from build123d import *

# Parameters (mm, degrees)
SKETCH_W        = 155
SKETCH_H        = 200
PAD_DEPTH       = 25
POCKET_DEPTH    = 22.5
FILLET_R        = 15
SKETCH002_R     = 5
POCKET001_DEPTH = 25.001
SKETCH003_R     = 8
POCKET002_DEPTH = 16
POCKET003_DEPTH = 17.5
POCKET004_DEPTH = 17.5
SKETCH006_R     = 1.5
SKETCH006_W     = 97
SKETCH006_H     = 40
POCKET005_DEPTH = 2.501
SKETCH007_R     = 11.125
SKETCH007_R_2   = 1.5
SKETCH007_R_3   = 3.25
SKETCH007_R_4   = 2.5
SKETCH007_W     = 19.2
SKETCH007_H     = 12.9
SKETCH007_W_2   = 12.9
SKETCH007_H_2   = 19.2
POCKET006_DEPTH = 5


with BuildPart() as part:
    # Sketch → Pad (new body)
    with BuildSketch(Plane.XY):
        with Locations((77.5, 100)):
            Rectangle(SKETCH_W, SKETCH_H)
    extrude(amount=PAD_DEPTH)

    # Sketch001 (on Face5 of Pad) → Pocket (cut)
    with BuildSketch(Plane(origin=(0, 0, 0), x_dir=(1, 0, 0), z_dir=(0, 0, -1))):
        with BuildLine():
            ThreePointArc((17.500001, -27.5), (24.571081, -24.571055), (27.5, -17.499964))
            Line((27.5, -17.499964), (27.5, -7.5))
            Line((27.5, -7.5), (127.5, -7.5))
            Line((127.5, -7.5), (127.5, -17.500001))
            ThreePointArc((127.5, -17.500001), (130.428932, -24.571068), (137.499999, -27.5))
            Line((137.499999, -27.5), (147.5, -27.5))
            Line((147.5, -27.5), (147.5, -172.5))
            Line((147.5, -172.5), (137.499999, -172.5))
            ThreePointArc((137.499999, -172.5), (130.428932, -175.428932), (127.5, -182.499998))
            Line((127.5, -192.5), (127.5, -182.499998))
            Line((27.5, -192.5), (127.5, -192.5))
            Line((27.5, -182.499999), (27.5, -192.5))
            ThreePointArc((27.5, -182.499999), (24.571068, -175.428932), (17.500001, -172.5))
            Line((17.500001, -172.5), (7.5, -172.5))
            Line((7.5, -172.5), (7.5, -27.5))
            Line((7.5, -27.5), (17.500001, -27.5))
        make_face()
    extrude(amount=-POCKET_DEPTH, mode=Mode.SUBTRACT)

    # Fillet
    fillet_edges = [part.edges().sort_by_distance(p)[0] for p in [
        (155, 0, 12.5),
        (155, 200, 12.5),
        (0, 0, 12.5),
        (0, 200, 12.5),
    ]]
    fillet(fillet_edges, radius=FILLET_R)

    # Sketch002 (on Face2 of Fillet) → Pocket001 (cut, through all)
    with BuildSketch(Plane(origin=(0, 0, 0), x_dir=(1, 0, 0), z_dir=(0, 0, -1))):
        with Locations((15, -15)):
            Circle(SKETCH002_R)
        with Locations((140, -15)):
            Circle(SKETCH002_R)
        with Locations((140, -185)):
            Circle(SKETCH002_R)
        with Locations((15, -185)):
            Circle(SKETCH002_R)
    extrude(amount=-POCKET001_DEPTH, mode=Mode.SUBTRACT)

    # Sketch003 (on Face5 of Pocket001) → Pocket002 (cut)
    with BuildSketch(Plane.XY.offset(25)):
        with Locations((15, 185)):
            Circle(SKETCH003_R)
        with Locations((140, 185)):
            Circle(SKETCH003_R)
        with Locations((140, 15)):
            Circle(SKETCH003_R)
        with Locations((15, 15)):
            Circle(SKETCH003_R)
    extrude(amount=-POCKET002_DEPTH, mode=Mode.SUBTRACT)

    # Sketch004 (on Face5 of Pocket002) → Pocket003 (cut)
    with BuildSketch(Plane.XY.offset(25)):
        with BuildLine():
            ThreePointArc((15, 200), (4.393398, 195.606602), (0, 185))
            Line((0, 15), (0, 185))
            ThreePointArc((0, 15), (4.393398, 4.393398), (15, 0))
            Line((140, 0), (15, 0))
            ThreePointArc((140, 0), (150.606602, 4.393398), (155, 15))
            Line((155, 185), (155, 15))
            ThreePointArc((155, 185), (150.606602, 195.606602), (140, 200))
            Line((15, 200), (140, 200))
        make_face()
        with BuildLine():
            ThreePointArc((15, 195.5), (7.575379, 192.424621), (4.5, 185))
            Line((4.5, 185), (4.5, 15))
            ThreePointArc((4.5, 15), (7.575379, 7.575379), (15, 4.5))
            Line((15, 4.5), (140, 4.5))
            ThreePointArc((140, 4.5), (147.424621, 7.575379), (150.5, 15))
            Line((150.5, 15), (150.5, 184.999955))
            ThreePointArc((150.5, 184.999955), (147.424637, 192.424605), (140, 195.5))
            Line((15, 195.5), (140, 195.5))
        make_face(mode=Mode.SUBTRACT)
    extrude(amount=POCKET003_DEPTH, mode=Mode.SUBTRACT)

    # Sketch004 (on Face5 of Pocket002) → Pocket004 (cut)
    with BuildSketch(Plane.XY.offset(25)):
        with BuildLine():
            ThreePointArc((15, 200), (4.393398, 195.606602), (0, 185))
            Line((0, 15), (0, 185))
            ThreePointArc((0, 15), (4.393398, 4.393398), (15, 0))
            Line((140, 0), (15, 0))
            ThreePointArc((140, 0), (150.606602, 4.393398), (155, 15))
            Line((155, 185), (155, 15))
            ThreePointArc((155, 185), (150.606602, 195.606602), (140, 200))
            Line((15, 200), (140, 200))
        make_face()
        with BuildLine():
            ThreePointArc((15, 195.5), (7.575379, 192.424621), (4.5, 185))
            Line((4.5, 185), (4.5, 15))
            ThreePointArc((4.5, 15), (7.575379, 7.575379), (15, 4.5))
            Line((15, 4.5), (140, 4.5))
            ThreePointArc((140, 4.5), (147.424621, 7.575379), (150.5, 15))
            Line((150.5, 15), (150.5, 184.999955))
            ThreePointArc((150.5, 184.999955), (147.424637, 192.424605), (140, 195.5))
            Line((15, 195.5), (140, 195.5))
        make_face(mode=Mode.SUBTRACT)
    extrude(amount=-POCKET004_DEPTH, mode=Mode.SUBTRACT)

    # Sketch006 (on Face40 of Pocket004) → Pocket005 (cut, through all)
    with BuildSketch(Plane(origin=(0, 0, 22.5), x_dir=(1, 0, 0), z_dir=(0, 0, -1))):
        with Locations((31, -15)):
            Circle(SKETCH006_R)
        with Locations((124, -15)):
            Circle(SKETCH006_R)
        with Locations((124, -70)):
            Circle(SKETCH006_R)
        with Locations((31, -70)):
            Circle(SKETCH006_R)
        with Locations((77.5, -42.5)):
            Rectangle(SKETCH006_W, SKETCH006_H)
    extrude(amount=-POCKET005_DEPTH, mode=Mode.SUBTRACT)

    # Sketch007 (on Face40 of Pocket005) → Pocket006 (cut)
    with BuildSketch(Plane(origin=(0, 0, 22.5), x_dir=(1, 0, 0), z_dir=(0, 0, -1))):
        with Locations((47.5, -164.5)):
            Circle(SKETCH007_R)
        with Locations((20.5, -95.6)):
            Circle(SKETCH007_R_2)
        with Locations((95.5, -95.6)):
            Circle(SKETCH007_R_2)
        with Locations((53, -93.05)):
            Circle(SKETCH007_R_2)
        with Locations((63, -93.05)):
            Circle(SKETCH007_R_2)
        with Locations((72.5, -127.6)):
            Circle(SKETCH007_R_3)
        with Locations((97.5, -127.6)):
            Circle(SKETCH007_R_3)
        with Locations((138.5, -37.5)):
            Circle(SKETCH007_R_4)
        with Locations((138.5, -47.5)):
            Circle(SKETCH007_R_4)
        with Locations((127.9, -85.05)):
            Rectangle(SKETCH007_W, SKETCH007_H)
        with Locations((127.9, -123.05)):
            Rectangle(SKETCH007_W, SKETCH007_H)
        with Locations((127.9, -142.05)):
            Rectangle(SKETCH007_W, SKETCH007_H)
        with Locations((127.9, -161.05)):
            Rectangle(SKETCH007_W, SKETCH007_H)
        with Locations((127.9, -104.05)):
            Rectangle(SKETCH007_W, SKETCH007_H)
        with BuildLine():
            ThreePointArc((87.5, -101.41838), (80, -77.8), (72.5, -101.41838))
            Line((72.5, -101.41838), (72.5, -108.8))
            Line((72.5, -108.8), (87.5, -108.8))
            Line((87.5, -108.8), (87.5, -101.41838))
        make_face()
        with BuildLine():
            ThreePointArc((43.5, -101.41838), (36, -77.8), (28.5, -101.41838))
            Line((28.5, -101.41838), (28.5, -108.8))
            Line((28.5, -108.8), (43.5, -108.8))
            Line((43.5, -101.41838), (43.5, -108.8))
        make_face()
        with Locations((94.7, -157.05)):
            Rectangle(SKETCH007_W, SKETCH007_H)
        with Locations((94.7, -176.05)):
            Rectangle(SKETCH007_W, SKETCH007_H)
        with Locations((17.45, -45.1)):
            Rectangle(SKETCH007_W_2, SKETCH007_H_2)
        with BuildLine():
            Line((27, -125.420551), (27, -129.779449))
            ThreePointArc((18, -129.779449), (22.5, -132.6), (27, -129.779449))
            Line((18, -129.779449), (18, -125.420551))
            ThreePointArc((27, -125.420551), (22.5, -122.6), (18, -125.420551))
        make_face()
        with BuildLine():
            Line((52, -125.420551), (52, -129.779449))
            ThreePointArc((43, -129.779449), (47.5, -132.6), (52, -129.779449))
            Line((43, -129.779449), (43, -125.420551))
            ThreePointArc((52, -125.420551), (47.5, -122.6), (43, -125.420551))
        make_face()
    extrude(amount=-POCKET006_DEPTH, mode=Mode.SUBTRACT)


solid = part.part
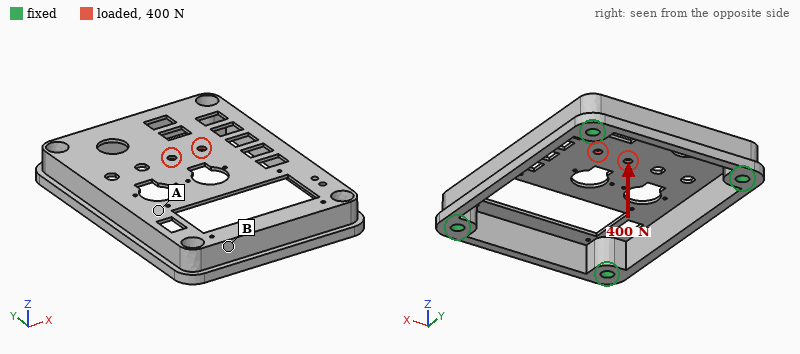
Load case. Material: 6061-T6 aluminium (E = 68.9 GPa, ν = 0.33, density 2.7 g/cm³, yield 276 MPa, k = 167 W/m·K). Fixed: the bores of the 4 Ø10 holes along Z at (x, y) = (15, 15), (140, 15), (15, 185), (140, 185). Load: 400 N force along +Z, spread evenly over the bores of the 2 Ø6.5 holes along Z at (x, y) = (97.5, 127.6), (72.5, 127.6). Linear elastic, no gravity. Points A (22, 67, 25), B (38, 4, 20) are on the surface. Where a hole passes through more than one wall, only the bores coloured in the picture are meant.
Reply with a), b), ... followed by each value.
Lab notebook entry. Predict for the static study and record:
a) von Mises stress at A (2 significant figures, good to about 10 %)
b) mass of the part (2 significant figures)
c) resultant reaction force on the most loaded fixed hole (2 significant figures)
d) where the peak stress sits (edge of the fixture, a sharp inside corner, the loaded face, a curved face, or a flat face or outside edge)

a) 22 MPa
b) 360 g
c) 210 N
d) the loaded face
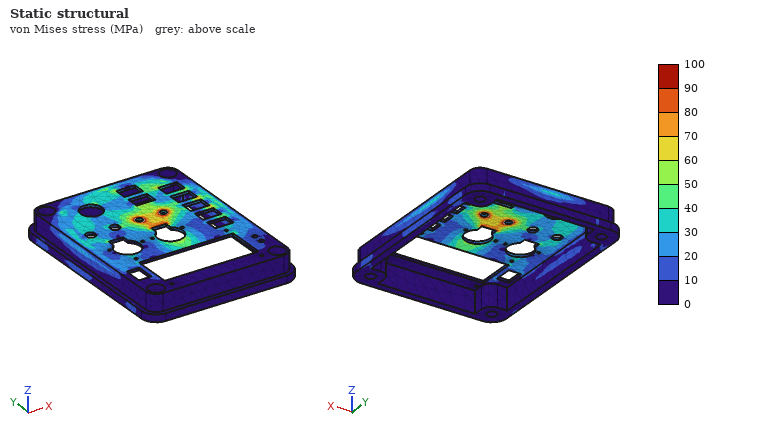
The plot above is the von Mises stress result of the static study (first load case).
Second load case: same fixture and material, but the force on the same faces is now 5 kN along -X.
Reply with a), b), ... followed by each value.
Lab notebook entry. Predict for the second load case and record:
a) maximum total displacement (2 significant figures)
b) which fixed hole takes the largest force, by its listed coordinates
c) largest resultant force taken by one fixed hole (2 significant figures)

a) 0.11 mm
b) (15, 185)
c) 2.5 kN
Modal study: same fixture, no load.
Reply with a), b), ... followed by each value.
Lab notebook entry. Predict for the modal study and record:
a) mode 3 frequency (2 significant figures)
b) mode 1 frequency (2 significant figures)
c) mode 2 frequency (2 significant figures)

a) 1600 Hz
b) 650 Hz
c) 1200 Hz
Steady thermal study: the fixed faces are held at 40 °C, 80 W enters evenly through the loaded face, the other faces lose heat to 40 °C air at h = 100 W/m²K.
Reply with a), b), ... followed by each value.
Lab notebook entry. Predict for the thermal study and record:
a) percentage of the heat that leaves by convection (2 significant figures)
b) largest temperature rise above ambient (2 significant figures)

a) 80 %
b) 71 K
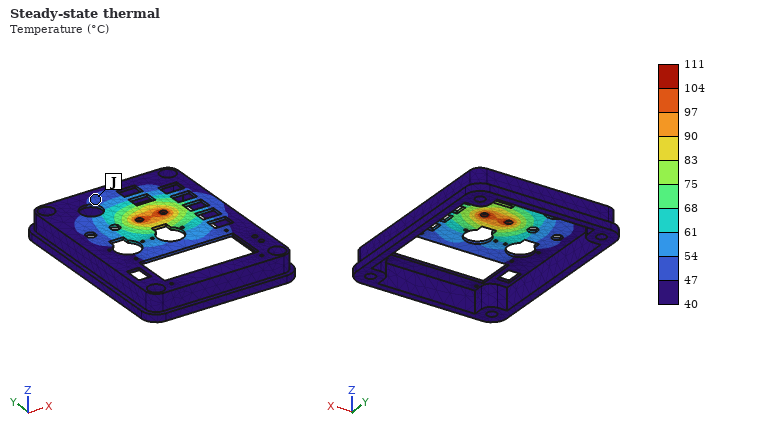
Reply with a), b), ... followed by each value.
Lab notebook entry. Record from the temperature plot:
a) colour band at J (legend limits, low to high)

a) 47 to 54 °C
